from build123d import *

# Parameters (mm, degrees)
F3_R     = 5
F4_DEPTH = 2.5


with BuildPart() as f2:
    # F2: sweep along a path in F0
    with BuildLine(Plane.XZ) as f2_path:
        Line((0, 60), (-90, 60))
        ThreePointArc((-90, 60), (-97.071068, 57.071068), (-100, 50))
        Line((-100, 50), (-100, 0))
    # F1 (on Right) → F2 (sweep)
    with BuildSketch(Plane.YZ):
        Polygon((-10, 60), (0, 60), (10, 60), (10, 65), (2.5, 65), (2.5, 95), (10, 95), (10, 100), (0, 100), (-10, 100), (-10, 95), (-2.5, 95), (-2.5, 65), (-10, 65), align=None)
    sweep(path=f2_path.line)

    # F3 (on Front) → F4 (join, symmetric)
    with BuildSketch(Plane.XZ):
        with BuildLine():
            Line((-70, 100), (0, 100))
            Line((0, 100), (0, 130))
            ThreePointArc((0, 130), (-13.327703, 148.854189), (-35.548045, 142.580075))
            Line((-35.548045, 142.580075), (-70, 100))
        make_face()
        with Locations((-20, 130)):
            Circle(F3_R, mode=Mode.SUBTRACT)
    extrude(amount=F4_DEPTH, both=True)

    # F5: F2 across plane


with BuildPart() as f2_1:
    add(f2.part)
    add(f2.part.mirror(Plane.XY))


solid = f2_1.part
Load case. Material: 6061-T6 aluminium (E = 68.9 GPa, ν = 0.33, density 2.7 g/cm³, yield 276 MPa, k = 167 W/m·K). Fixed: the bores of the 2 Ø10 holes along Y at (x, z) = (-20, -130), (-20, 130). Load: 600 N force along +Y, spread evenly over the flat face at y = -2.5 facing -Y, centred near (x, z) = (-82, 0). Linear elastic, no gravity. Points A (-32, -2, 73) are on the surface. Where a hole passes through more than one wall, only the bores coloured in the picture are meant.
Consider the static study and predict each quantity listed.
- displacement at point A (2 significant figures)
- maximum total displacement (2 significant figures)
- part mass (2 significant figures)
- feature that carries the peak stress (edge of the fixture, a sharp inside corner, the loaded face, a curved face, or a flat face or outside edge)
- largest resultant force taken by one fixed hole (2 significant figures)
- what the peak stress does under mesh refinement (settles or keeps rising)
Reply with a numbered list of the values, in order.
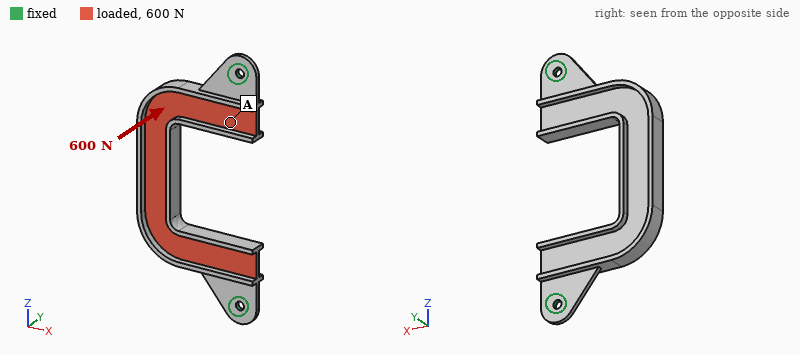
1. 0.26 mm
2. 1.3 mm
3. 420 g
4. edge of the fixture
5. 300 N
6. keeps rising
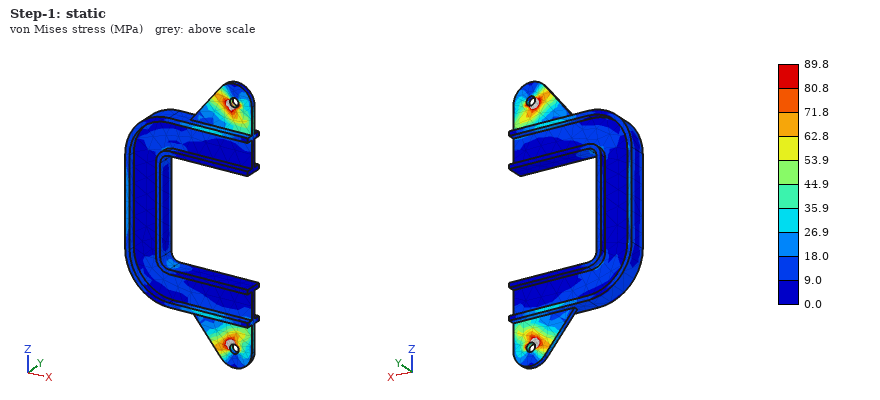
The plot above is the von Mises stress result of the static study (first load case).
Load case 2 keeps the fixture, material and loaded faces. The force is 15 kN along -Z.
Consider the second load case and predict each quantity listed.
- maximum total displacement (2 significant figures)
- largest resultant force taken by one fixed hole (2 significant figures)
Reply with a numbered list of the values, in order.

1. 0.38 mm
2. 8.1 kN
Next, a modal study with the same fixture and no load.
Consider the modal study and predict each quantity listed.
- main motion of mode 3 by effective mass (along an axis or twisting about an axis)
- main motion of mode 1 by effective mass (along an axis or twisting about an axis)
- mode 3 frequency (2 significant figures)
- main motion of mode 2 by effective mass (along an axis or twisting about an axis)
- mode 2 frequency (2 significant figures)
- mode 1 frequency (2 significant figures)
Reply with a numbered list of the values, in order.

1. along Y
2. along Y
3. 830 Hz
4. twisting about X
5. 580 Hz
6. 210 Hz
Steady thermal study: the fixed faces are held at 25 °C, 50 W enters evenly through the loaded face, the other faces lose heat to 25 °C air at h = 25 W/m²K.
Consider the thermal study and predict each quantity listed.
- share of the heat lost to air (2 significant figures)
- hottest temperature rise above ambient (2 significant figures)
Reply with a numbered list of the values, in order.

1. 46 %
2. 25 K
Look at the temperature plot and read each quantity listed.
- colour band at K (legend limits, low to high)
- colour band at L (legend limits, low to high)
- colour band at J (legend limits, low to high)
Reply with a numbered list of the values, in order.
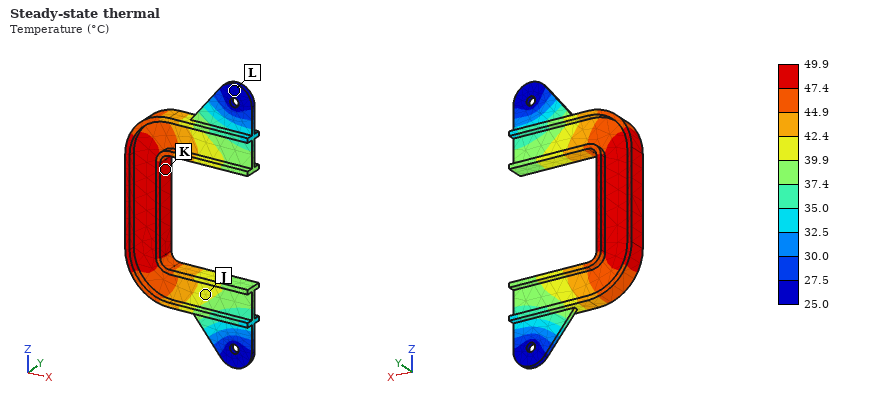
1. 47.4 to 49.9 °C
2. 25.0 to 27.5 °C
3. 39.9 to 42.4 °C
